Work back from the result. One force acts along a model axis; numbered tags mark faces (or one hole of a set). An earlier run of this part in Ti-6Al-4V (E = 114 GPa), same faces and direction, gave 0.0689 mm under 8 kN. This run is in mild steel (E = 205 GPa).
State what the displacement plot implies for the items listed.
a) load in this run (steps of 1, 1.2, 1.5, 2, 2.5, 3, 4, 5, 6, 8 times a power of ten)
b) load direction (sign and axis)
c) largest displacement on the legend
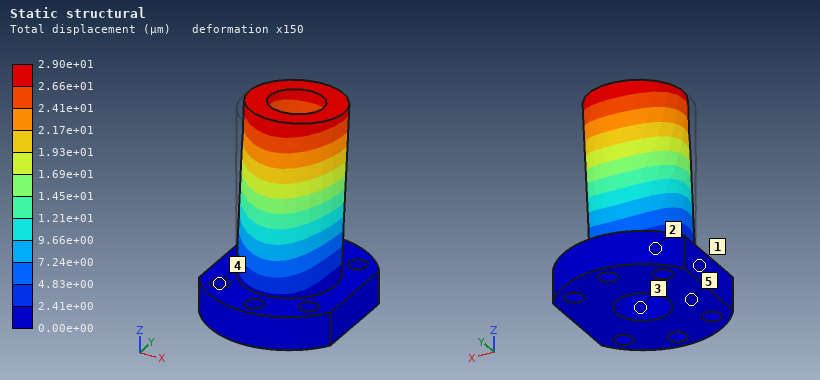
6 kN
+Y
2.90e+01 µm
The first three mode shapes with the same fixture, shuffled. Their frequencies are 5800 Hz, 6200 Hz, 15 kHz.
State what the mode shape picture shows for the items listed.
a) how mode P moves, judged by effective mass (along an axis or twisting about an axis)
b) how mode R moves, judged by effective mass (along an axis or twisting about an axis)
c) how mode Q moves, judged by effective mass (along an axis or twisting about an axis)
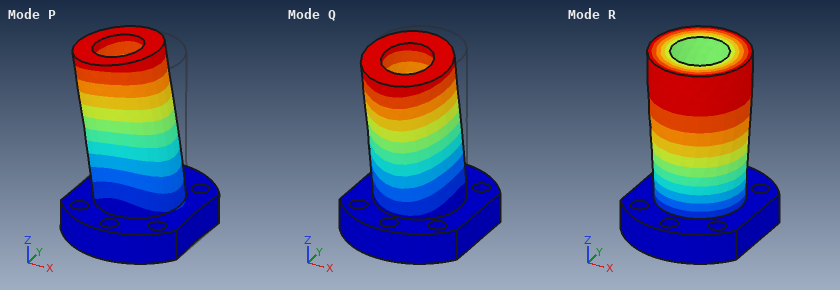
along X
twisting about Z
along Y
